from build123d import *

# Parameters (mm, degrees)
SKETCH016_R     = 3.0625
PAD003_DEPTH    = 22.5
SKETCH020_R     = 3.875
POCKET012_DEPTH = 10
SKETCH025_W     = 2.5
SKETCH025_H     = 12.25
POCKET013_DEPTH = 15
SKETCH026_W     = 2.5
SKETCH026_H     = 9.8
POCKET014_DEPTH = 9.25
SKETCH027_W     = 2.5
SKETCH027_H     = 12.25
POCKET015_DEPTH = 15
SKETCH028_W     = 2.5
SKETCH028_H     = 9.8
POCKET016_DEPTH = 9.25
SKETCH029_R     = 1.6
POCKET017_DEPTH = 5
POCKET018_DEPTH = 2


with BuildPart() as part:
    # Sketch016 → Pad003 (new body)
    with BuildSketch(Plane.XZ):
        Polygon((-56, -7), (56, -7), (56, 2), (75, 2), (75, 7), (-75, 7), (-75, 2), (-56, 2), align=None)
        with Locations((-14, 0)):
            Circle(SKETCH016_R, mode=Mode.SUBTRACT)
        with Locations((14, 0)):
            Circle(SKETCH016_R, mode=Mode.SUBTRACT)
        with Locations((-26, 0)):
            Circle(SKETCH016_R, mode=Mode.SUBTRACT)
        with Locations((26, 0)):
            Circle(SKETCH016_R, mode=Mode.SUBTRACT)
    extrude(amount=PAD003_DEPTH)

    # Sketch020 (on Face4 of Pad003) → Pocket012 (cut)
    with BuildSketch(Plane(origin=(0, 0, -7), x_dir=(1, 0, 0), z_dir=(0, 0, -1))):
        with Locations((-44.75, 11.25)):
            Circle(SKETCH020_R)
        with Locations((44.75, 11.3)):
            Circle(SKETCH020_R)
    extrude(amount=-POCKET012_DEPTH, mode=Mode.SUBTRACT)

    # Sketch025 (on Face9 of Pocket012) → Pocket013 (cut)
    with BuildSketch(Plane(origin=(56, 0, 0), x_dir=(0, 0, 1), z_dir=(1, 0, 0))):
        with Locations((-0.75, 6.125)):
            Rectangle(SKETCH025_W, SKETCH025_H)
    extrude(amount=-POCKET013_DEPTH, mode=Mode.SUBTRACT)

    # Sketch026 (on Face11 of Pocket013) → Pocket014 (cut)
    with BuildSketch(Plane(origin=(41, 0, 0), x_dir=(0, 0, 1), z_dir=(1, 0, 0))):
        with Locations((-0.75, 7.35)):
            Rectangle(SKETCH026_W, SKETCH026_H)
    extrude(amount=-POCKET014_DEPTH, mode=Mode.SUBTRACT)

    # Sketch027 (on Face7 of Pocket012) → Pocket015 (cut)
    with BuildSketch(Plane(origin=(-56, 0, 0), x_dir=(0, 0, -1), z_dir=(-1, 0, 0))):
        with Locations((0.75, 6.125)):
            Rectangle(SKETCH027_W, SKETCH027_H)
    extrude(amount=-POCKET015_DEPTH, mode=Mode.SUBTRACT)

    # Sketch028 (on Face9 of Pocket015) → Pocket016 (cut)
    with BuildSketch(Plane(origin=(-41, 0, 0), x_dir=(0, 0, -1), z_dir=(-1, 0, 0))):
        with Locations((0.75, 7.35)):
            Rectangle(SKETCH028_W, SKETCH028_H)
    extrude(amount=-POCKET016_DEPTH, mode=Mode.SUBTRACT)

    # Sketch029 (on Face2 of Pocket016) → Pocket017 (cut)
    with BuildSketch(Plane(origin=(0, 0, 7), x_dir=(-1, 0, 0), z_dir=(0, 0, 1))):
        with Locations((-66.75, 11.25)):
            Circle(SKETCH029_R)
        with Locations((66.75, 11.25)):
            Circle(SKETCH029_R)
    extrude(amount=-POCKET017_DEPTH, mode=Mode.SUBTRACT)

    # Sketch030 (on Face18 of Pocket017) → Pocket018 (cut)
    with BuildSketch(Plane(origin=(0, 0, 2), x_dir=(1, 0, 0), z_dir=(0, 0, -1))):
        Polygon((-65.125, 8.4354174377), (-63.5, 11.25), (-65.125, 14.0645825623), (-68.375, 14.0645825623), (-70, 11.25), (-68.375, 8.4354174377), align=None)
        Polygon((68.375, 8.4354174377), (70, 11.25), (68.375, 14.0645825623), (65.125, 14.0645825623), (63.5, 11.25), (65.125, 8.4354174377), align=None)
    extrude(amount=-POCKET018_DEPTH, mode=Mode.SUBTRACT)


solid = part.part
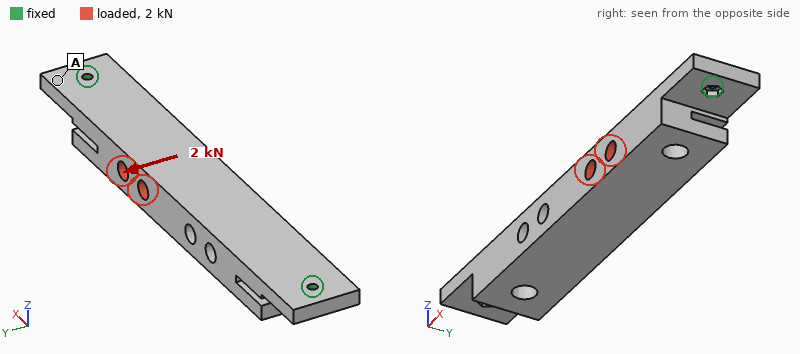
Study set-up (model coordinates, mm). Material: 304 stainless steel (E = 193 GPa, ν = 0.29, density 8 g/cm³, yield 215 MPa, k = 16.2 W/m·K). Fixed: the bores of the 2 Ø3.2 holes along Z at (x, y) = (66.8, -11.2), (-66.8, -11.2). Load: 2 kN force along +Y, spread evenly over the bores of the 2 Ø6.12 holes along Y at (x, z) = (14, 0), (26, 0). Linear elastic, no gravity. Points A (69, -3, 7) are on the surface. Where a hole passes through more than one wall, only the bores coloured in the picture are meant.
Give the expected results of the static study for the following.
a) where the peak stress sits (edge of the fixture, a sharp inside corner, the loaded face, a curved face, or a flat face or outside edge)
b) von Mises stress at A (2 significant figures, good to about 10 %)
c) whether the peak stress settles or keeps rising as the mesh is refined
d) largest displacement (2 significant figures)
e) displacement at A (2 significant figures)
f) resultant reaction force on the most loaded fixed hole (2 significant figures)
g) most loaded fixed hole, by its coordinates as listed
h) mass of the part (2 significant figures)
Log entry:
edge of the fixture
29 MPa
keeps rising
71 µm
13 µm
1.3 kN
(66.8, -11.2)
280 g
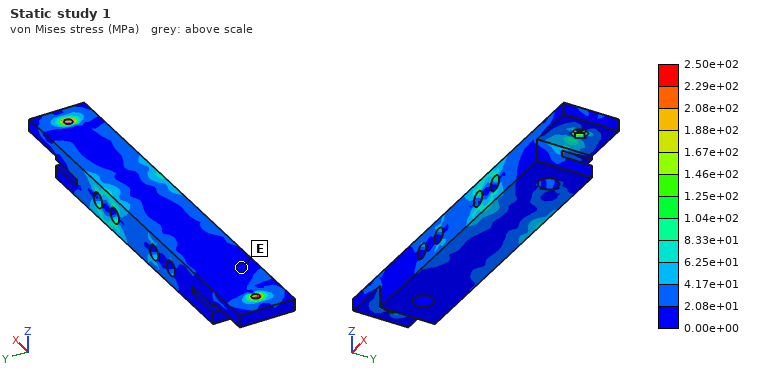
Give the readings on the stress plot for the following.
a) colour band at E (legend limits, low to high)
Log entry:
0.00e+00 to 2.08e+01 MPa
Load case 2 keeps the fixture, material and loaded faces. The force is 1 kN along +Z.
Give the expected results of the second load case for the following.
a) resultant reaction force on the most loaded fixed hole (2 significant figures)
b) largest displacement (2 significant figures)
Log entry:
1.4 kN
35 µm
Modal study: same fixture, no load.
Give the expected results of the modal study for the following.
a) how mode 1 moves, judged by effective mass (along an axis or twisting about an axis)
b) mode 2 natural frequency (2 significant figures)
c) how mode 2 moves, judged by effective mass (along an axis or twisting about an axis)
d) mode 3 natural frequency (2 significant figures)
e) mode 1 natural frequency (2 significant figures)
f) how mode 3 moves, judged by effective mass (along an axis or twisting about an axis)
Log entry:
along Y
2200 Hz
along Z
3600 Hz
2100 Hz
along Y
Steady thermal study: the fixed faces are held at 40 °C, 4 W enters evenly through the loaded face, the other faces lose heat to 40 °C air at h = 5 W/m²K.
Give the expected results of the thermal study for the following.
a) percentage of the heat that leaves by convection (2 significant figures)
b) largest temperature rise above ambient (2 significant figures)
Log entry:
32 %
34 K
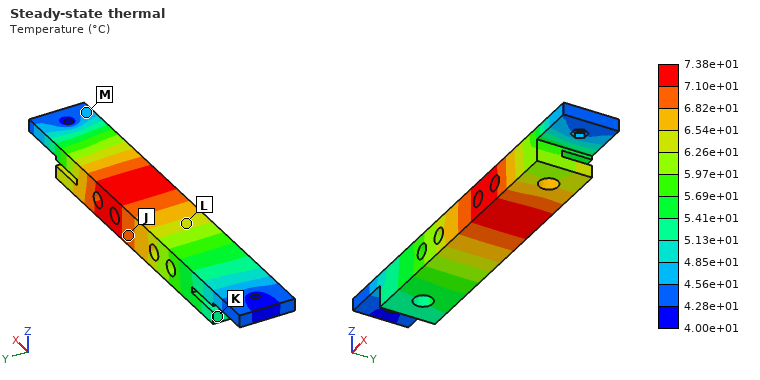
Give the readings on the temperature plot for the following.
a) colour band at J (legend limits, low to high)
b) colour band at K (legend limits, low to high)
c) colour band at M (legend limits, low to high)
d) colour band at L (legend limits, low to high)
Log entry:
6.82e+01 to 7.10e+01 °C
5.13e+01 to 5.41e+01 °C
4.56e+01 to 4.85e+01 °C
6.26e+01 to 6.54e+01 °C
